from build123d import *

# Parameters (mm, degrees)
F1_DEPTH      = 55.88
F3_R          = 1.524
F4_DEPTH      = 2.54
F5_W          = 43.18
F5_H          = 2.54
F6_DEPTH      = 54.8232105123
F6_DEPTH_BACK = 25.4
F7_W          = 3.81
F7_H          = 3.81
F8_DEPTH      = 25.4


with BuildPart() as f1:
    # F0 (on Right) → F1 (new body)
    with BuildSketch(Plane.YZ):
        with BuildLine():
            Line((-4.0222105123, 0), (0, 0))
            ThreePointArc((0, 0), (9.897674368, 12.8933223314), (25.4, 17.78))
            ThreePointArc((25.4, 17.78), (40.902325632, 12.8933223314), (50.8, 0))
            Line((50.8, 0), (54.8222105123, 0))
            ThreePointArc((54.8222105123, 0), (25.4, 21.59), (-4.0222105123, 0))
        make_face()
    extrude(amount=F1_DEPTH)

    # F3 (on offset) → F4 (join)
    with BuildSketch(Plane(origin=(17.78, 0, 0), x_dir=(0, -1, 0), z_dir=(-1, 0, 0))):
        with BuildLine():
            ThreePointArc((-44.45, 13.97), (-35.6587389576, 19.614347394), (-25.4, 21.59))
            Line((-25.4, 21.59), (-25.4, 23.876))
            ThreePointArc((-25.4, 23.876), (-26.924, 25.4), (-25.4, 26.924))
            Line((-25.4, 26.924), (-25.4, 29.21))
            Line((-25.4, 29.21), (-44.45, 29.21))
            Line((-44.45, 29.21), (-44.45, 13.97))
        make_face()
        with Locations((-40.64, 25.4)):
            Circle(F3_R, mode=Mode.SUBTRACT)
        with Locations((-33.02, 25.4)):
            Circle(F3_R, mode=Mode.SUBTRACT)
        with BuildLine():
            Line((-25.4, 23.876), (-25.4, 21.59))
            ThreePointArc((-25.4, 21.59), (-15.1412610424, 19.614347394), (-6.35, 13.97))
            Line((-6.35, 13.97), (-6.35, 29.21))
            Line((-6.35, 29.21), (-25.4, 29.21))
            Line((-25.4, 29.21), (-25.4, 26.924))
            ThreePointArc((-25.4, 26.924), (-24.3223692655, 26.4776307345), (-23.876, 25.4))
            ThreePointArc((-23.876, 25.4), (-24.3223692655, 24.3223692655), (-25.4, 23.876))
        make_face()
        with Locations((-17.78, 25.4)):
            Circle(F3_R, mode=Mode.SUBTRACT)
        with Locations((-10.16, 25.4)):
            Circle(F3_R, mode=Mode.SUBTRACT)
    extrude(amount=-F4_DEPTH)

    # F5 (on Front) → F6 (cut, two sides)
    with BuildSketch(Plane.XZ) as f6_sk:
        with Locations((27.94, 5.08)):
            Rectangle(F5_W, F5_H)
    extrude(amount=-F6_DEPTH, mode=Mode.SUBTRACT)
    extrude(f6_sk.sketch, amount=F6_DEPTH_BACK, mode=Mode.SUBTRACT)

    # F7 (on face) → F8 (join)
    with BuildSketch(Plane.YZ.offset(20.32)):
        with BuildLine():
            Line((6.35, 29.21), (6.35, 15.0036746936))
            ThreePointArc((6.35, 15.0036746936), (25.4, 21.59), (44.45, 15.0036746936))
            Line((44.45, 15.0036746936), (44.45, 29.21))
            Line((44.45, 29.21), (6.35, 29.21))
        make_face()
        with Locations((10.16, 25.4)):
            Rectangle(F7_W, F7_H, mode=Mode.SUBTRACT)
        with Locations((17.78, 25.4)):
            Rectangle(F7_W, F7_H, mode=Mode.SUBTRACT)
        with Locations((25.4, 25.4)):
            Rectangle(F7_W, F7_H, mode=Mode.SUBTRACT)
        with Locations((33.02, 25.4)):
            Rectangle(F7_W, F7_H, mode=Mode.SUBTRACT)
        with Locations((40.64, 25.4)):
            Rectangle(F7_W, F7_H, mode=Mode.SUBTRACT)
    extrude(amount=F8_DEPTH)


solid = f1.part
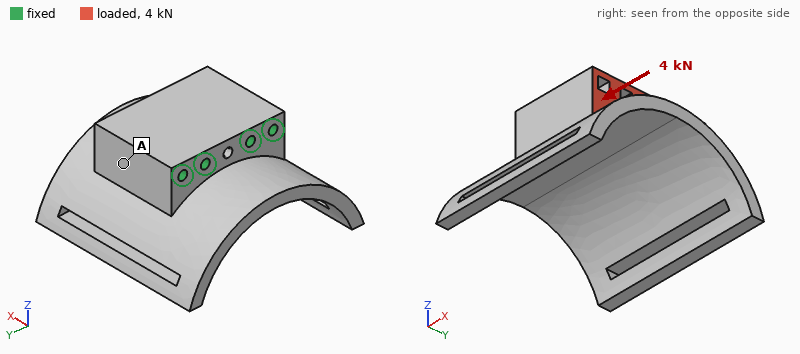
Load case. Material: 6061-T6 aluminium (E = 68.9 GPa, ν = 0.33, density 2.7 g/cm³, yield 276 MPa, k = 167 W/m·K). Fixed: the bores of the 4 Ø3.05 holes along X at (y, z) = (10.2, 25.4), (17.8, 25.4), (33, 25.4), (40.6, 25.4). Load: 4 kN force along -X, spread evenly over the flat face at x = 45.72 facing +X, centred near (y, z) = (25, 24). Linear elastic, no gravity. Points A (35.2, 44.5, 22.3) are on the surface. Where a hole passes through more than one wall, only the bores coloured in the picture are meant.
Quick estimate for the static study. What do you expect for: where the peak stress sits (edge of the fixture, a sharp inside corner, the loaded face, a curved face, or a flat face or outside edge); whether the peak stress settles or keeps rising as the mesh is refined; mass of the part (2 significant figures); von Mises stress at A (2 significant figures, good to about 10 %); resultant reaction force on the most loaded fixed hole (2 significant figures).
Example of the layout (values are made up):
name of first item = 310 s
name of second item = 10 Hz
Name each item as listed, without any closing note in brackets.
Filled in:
where the peak stress sits = edge of the fixture
whether the peak stress settles or keeps rising as the mesh is refined = keeps rising
mass of the part = 62 g
von Mises stress at A = 12 MPa
resultant reaction force on the most loaded fixed hole = 1.1 kN
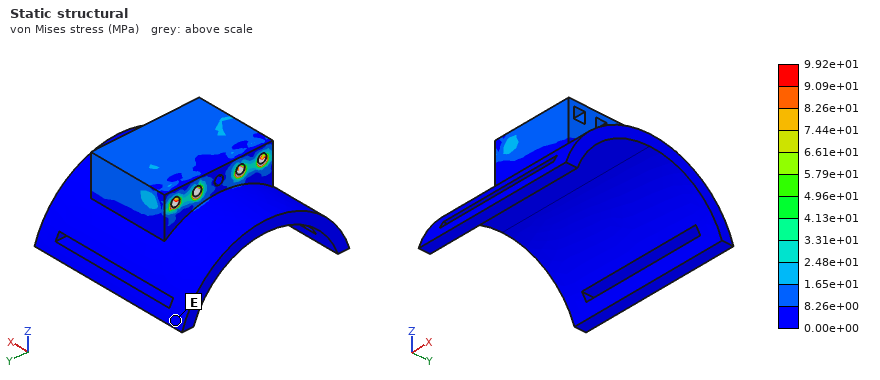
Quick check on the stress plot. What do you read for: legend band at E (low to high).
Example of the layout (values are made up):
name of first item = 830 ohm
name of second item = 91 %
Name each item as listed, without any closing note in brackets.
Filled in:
legend band at E = 0.00e+00 to 8.26e+00 MPa
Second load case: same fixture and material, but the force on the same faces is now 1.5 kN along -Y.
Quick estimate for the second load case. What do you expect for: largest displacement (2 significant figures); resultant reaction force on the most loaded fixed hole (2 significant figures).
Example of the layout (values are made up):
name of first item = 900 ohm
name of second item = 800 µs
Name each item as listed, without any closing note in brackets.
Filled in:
largest displacement = 21 µm
resultant reaction force on the most loaded fixed hole = 1.1 kN
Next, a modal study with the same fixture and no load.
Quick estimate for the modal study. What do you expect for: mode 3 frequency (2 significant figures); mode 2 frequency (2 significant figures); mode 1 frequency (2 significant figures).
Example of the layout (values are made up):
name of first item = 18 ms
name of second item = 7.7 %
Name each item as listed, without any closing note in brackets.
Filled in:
mode 3 frequency = 4500 Hz
mode 2 frequency = 4300 Hz
mode 1 frequency = 2200 Hz
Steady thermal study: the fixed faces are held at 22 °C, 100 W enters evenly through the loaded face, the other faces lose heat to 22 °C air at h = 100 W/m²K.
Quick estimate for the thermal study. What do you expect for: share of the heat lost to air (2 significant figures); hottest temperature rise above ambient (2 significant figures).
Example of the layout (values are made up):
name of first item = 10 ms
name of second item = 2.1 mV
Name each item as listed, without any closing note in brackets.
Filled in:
share of the heat lost to air = 23 %
hottest temperature rise above ambient = 41 K
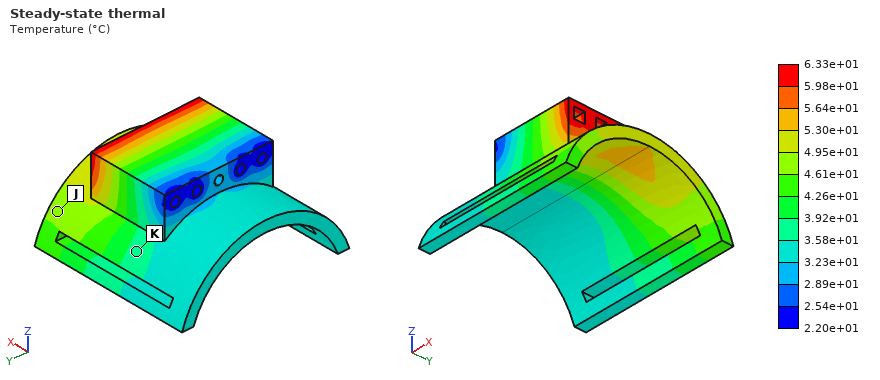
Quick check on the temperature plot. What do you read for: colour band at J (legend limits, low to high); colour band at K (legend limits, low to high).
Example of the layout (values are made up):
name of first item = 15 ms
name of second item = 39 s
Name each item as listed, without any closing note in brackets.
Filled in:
colour band at J = 4.61e+01 to 4.95e+01 °C
colour band at K = 3.58e+01 to 3.92e+01 °C
